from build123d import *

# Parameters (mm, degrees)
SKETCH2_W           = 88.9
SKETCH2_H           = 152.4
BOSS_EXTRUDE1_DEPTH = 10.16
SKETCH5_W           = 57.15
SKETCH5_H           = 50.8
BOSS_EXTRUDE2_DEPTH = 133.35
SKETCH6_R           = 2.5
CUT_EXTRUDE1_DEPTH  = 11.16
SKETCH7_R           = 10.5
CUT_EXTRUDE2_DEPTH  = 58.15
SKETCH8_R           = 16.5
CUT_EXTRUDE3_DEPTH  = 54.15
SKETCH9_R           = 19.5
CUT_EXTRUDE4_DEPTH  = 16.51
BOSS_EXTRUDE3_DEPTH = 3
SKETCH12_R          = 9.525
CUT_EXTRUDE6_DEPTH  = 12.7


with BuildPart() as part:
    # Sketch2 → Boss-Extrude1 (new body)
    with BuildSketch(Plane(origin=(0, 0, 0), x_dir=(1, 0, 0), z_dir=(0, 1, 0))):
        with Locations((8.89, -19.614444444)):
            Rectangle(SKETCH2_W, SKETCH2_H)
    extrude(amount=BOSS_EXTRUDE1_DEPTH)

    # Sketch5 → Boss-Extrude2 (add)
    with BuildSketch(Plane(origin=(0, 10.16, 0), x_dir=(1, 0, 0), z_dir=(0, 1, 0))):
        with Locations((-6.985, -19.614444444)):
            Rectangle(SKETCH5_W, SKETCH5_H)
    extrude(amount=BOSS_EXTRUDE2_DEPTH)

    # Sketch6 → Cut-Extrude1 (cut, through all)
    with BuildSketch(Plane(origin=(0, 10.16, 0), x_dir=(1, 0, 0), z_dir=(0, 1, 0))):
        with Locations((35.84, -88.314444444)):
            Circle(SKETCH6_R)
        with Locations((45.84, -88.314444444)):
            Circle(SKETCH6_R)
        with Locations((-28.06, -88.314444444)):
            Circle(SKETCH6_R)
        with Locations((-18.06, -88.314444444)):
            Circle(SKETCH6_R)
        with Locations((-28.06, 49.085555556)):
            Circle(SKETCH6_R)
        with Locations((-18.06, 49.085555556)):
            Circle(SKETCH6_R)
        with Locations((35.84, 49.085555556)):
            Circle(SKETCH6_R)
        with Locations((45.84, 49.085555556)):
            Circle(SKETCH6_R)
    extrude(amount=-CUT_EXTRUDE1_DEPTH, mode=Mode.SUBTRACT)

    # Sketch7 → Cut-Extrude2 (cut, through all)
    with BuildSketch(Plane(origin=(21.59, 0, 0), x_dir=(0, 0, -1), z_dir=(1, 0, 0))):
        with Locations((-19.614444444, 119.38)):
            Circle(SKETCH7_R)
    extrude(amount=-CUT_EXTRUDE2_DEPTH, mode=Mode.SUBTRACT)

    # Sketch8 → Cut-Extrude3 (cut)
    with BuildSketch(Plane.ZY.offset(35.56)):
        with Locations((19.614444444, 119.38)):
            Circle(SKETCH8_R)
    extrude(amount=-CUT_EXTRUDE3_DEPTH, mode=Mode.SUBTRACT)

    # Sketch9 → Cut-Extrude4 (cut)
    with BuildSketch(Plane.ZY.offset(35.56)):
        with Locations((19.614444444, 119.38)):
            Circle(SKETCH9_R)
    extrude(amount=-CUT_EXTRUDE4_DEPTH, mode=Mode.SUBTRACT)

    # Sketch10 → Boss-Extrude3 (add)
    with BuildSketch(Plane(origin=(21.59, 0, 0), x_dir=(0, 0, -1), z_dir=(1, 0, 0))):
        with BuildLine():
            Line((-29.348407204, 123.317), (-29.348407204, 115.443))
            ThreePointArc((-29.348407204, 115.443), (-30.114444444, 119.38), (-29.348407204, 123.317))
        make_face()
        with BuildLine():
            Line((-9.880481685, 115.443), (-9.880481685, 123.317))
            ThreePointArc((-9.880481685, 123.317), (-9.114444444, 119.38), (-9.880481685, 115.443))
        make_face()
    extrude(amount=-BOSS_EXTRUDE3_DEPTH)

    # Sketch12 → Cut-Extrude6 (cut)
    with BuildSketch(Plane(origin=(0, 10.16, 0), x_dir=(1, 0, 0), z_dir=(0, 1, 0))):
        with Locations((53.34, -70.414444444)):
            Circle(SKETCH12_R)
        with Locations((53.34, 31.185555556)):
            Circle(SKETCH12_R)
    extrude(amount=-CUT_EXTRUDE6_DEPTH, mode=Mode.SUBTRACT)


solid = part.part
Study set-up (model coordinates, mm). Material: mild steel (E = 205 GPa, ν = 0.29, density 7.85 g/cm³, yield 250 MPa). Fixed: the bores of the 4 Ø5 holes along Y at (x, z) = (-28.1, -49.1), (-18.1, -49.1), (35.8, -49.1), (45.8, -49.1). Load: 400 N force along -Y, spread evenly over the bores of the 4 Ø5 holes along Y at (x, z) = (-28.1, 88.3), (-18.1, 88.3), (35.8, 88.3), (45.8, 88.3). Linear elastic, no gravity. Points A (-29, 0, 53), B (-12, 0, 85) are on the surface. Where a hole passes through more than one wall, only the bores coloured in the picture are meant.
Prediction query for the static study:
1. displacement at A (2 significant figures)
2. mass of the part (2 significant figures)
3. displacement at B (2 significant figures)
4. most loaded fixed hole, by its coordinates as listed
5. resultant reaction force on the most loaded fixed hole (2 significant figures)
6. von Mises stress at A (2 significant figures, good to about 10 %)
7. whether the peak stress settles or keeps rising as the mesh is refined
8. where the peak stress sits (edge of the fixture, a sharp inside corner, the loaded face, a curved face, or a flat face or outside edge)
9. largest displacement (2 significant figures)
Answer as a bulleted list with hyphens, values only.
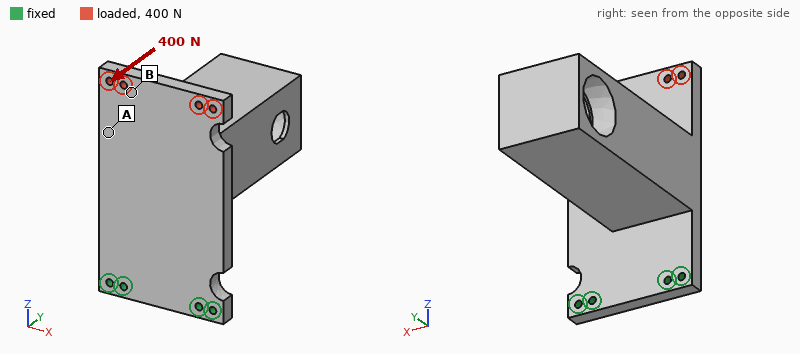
- 0.13 mm
- 3.7 kg
- 0.19 mm
- (-18.1, -49.1)
- 170 N
- 10 MPa
- keeps rising
- edge of the fixture
- 0.26 mm
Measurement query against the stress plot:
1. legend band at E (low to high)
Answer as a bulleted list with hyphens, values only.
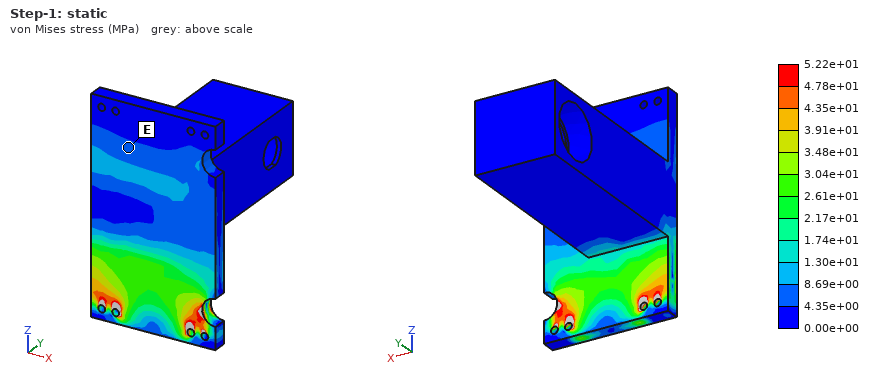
- 4.35e+00 to 8.69e+00 MPa
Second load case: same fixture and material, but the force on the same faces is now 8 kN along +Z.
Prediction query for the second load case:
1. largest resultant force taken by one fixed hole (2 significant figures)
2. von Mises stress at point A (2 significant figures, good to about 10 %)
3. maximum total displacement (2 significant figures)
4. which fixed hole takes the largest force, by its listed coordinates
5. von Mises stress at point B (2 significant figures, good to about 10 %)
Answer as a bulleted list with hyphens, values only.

- 3.1 kN
- 11 MPa
- 15 µm
- (35.8, -49.1)
- 15 MPa
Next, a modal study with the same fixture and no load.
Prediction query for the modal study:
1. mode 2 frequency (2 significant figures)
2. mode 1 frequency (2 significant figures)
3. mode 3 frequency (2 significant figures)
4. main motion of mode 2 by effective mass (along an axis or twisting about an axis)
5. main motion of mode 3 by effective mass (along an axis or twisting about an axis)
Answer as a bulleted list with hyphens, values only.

- 390 Hz
- 170 Hz
- 1100 Hz
- along X
- along Y
